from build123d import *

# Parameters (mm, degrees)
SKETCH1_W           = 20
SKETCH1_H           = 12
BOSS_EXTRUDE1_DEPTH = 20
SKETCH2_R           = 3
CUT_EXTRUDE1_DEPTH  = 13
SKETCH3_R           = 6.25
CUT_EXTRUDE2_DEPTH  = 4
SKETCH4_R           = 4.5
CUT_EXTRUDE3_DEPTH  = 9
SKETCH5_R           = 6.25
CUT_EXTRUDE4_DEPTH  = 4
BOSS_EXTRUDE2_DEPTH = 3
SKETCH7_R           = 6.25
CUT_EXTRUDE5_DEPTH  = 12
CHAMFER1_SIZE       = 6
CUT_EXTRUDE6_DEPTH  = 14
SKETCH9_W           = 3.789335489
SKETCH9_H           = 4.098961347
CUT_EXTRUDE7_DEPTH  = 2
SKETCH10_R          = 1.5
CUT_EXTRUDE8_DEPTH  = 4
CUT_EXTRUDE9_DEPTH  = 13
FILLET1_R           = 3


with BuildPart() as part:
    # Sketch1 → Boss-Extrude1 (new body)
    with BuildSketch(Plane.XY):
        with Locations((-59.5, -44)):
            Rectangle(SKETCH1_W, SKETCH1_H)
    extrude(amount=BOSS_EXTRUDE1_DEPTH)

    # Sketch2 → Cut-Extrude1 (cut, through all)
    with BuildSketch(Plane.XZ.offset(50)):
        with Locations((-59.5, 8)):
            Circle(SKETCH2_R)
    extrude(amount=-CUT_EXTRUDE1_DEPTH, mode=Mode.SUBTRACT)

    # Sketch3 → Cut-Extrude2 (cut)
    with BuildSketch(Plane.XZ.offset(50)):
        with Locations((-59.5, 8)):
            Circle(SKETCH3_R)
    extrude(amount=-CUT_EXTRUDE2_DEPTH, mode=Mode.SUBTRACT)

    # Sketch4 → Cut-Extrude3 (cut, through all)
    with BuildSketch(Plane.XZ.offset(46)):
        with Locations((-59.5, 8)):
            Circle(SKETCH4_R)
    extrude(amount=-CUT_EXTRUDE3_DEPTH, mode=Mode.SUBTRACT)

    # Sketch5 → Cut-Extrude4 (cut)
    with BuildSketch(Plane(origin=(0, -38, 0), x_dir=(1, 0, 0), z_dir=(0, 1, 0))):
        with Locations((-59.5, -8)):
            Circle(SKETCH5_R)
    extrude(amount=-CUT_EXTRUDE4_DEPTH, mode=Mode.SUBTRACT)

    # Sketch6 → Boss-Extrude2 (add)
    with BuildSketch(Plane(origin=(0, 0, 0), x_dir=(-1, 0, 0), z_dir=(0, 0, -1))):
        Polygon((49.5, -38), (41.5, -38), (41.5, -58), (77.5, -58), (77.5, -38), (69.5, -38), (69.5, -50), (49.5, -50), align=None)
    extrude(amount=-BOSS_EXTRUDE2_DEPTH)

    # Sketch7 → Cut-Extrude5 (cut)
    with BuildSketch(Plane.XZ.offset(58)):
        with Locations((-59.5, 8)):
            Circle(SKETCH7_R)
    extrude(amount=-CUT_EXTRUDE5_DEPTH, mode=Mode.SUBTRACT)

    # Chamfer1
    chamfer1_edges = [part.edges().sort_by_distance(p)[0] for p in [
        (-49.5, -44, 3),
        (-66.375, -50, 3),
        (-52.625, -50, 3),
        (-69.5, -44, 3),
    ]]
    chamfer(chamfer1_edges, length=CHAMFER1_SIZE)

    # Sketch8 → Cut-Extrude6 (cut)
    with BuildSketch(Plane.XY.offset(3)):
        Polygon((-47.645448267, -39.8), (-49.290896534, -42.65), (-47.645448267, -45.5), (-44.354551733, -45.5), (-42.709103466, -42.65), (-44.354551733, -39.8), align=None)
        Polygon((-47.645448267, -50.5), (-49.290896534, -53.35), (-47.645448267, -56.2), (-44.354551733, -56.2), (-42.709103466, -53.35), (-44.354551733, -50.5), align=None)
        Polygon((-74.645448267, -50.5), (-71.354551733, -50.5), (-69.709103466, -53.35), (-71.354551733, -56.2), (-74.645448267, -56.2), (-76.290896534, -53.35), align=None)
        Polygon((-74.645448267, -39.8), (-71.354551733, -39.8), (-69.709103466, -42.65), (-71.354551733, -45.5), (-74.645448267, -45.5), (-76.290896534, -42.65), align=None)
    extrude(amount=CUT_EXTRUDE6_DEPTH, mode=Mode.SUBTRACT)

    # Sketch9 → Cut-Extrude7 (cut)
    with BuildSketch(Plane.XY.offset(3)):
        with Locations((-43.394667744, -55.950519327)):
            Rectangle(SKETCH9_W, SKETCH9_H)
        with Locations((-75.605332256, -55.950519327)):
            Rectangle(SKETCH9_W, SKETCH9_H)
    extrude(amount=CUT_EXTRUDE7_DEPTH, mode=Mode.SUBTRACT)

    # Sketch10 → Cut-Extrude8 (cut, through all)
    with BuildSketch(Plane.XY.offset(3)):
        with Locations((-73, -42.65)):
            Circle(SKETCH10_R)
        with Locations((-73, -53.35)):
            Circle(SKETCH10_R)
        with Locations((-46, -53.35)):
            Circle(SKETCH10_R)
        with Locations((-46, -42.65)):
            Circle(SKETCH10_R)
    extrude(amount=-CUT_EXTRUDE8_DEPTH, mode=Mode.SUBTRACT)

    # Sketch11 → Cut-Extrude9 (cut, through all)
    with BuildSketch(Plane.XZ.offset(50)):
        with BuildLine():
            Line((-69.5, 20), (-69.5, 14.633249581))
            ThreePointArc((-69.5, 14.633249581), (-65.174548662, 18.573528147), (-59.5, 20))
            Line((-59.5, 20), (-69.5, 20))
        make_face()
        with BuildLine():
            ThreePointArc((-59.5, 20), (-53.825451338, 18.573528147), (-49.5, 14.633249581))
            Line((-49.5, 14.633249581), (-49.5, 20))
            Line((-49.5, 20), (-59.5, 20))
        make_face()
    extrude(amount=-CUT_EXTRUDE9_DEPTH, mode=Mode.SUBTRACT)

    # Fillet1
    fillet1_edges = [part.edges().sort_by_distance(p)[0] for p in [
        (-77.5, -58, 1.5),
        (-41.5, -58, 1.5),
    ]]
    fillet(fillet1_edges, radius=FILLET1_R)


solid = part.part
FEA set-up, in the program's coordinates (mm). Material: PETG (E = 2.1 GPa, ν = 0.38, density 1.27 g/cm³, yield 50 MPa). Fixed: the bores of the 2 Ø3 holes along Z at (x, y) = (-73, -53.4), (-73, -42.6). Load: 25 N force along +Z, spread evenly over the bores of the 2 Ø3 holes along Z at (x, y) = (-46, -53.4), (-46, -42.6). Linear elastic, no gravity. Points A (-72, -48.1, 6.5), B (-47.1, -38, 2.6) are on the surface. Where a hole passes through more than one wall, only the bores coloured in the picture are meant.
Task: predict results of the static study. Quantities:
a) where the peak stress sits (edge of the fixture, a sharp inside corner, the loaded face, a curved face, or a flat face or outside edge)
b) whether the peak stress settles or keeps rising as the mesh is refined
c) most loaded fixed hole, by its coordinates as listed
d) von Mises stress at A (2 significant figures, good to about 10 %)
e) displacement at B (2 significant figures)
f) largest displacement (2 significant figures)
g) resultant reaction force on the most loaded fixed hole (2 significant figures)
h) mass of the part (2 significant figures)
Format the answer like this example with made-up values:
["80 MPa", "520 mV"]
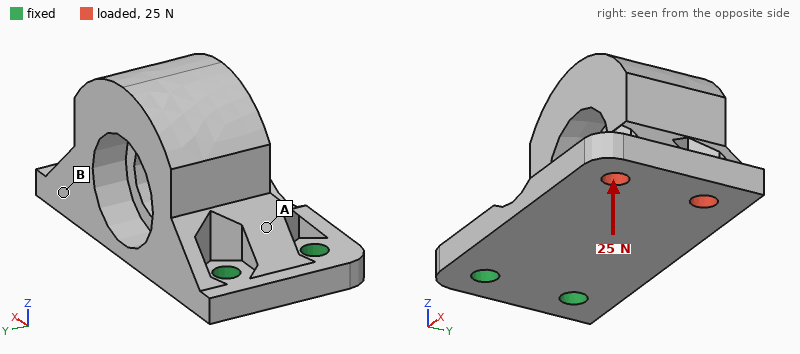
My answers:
["edge of the fixture", "keeps rising", "(-73, -42.6)", "5.8 MPa", "0.39 mm", "0.51 mm", "16 N", "6.3 g"]
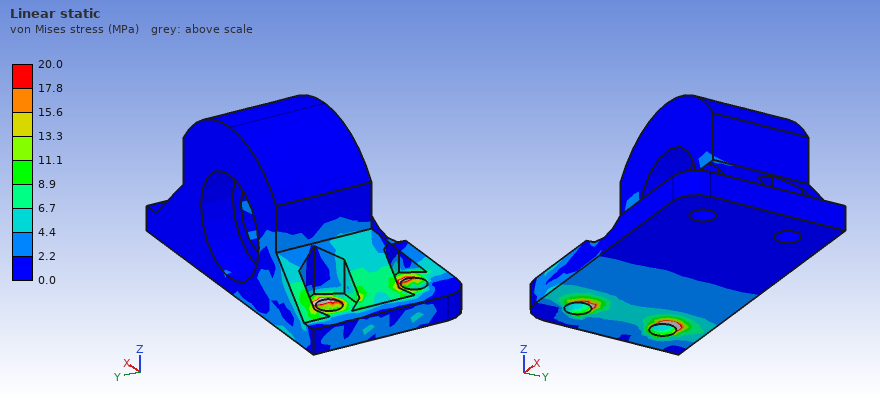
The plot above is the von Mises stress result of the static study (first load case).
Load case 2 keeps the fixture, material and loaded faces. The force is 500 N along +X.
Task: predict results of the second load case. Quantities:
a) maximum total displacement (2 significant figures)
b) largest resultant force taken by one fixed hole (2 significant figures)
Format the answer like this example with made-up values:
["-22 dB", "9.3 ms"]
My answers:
["0.23 mm", "250 N"]
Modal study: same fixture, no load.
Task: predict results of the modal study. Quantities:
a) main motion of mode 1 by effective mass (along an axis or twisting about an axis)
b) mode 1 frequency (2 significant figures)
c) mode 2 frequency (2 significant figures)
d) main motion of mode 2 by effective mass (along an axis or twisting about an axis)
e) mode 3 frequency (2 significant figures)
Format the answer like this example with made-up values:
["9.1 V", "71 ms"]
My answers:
["along Z", "760 Hz", "2100 Hz", "along Y", "2900 Hz"]
